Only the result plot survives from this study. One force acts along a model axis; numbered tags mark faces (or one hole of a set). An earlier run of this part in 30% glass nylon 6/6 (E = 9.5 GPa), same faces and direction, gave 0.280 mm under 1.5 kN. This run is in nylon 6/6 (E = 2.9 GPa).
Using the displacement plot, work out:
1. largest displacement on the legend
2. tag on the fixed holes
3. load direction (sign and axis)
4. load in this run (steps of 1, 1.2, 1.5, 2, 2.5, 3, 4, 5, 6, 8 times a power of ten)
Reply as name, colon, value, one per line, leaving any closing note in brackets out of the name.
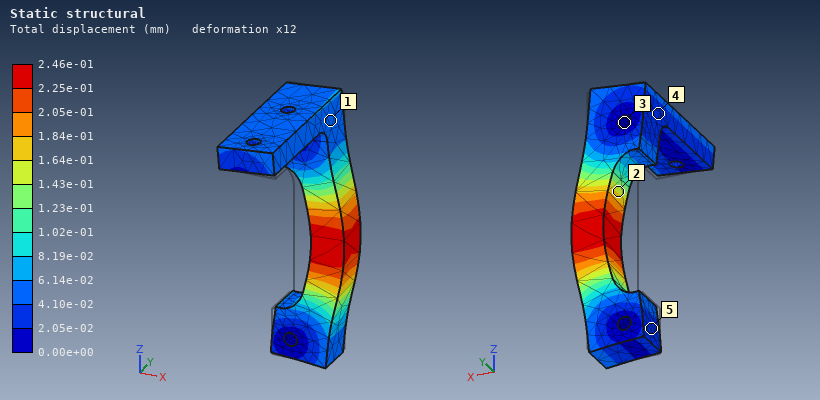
largest displacement on the legend: 2.46e-01 mm
tag on the fixed holes: 3
load direction: +X
load in this run: 400 N
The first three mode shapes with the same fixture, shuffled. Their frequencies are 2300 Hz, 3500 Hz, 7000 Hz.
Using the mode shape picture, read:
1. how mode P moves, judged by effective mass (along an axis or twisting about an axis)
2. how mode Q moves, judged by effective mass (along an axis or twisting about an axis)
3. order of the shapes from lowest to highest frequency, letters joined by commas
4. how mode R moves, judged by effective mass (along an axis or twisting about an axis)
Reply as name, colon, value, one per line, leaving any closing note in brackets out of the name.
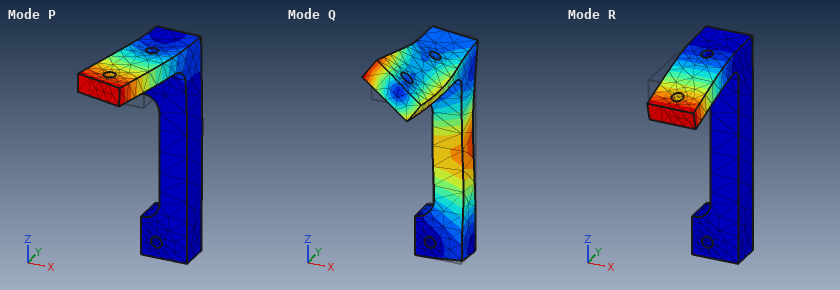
how mode P moves, judged by effective mass: along X
how mode Q moves, judged by effective mass: along Y
order of the shapes from lowest to highest frequency, letters joined by commas: R, P, Q
how mode R moves, judged by effective mass: along Z
